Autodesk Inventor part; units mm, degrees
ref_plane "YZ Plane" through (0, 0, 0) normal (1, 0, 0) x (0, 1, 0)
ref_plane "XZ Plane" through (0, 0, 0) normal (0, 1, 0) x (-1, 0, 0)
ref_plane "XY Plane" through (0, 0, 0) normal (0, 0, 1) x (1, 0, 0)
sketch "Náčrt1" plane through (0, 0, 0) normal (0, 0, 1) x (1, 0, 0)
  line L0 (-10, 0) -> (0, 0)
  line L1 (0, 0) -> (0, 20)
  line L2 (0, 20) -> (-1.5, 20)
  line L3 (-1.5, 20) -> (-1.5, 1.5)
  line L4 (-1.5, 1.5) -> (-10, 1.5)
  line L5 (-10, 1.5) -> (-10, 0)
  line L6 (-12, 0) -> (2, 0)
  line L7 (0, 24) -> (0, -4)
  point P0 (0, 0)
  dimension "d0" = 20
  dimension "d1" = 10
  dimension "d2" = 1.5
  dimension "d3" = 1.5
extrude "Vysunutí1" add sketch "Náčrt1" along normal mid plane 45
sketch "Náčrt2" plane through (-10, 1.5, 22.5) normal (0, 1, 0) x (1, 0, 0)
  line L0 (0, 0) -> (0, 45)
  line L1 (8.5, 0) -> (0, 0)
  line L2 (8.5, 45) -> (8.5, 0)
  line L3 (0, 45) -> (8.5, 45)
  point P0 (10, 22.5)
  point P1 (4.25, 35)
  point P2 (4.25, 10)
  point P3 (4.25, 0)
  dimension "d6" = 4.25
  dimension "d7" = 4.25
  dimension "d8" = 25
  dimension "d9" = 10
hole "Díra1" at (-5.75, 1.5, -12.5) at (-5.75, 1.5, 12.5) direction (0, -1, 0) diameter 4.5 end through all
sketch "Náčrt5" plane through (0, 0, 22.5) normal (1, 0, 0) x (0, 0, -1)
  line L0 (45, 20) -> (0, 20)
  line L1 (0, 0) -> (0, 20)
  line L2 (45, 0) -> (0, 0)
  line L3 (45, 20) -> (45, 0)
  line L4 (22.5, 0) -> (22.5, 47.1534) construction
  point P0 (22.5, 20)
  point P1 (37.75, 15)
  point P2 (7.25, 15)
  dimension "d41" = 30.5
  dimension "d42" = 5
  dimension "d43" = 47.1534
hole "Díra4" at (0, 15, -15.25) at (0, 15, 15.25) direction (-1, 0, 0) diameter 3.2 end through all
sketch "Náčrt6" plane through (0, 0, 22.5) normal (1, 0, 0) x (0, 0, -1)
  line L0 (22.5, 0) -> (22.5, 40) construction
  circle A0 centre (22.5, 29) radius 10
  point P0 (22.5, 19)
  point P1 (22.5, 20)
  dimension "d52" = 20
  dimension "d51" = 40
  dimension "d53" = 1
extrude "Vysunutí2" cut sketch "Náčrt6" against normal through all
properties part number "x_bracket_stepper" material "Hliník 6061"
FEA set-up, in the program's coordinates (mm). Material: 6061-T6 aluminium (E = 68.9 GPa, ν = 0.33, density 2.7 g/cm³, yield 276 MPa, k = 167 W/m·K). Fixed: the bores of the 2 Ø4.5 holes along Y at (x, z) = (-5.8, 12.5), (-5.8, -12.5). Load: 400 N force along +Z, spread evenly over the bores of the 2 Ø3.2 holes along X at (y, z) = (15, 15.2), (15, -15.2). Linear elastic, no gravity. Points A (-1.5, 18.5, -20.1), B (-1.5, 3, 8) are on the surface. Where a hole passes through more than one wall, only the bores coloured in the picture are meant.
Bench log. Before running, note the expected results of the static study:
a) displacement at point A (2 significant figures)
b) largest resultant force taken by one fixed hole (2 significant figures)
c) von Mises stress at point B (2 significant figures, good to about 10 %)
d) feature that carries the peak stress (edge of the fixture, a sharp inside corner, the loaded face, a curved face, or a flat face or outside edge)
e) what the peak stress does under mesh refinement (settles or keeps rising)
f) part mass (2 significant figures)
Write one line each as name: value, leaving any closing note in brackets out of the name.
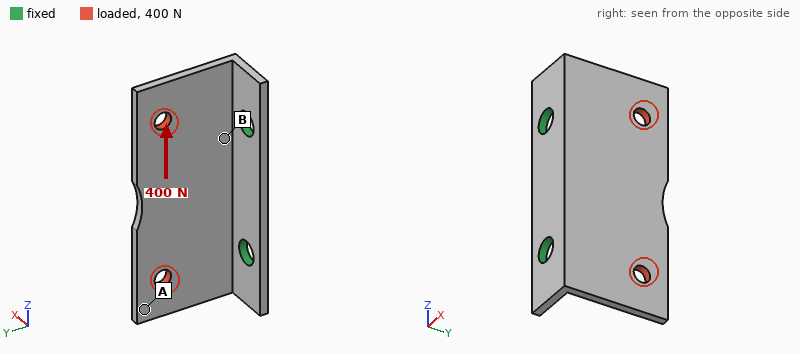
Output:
displacement at point A: 57 µm
largest resultant force taken by one fixed hole: 300 N
von Mises stress at point B: 37 MPa
feature that carries the peak stress: edge of the fixture
what the peak stress does under mesh refinement: keeps rising
part mass: 5.0 g
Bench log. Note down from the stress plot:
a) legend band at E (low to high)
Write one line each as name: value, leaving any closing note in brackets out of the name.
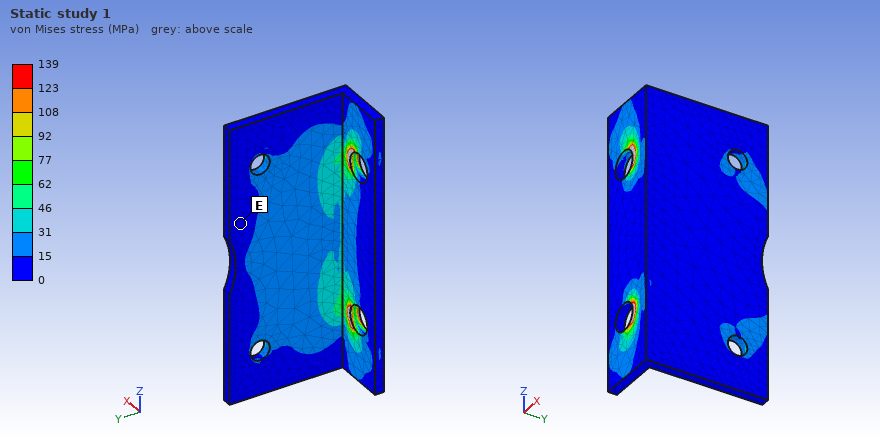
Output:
legend band at E: 0 to 15 MPa
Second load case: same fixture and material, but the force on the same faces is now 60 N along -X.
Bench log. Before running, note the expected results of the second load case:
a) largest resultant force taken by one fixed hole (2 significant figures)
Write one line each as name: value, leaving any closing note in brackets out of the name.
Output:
largest resultant force taken by one fixed hole: 30 N
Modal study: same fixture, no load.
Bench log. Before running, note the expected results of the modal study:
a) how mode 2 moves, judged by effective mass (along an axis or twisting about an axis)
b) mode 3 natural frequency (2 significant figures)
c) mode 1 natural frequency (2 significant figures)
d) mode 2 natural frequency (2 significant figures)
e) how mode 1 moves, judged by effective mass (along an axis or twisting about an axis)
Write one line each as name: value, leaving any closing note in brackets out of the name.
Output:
how mode 2 moves, judged by effective mass: twisting about Y
mode 3 natural frequency: 7600 Hz
mode 1 natural frequency: 2600 Hz
mode 2 natural frequency: 3900 Hz
how mode 1 moves, judged by effective mass: along X
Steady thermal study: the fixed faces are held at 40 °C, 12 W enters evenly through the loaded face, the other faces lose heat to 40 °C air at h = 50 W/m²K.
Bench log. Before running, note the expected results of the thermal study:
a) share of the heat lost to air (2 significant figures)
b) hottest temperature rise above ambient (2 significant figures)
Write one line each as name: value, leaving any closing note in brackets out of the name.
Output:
share of the heat lost to air: 12 %
hottest temperature rise above ambient: 26 K
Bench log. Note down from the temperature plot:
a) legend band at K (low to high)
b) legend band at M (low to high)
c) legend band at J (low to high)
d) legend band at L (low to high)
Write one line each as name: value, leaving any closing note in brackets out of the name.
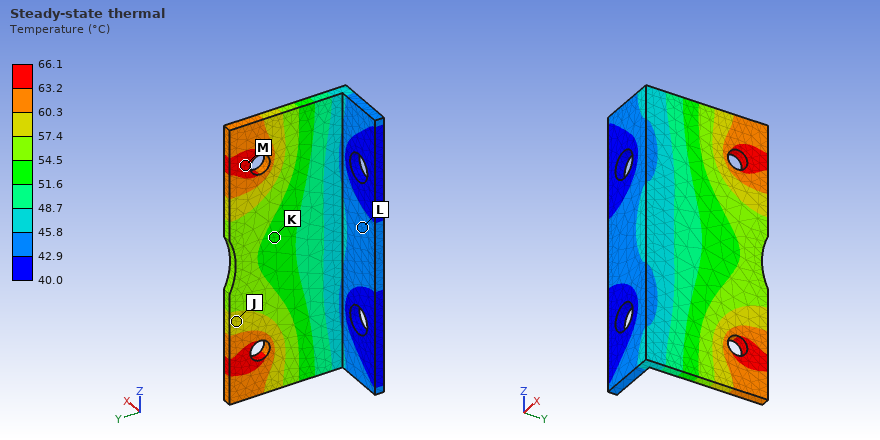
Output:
legend band at K: 51.6 to 54.5 °C
legend band at M: 63.2 to 66.1 °C
legend band at J: 57.4 to 60.3 °C
legend band at L: 42.9 to 45.8 °C
